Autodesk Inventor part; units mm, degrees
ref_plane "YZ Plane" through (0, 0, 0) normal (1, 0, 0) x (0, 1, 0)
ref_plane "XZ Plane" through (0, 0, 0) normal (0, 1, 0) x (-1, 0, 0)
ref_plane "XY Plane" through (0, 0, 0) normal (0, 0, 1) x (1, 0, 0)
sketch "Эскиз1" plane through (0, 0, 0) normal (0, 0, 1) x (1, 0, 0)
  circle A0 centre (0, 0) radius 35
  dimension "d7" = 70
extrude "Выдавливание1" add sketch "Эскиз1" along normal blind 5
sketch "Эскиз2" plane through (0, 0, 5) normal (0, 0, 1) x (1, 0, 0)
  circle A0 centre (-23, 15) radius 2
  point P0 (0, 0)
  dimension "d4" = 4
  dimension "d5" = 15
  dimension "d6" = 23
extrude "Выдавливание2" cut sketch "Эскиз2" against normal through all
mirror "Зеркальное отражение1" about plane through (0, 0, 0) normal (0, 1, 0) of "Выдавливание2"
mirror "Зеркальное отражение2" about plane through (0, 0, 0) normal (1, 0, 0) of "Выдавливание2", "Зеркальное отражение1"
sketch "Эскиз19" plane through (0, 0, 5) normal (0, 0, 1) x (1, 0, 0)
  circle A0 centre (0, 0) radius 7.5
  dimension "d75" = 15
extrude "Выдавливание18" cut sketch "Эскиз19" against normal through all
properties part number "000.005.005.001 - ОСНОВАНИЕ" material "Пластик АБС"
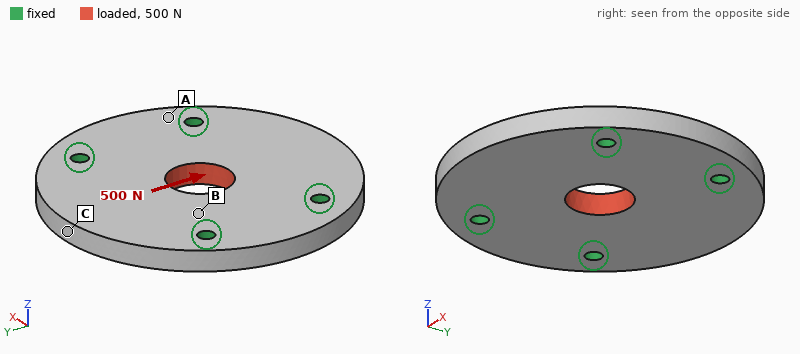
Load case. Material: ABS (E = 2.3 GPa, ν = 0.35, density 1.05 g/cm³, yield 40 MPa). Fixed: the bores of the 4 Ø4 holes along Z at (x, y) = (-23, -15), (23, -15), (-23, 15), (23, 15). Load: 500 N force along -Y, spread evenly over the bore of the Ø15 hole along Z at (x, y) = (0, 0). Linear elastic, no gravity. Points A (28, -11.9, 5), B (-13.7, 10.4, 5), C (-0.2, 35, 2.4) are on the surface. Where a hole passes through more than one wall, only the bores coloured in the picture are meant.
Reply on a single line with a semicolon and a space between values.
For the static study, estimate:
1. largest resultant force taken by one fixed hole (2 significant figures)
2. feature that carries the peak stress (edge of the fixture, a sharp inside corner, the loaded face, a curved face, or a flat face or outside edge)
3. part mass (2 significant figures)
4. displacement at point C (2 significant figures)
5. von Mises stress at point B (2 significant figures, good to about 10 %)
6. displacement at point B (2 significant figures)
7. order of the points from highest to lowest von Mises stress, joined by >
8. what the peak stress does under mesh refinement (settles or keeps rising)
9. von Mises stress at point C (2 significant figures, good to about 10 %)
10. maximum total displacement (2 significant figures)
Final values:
130 N; edge of the fixture; 19 g; 16 µm; 1.8 MPa; 13 µm; B > C > A; keeps rising; 1.1 MPa; 28 µm
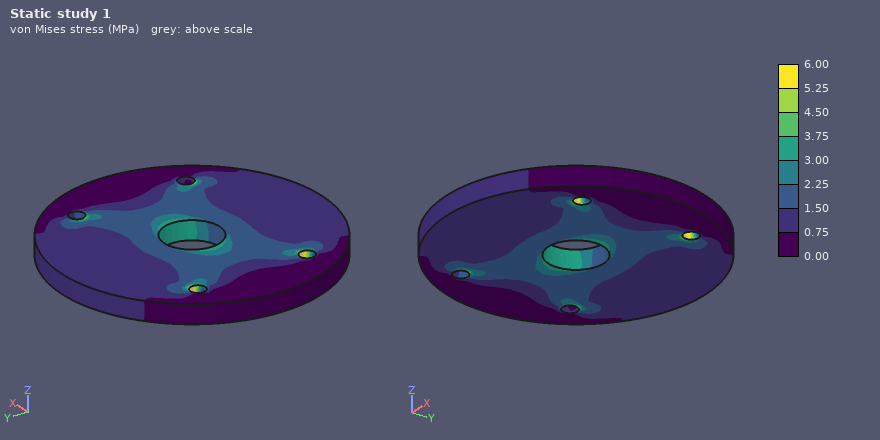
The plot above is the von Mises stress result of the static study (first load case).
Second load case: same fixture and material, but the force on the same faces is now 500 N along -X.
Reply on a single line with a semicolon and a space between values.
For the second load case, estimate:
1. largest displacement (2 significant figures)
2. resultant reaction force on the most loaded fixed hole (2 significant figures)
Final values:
19 µm; 130 N
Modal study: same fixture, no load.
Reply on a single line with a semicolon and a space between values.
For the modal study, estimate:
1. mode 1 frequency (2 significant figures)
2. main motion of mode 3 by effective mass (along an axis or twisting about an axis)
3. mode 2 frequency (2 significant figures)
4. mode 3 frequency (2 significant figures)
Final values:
2300 Hz; along Z; 2300 Hz; 3600 Hz
